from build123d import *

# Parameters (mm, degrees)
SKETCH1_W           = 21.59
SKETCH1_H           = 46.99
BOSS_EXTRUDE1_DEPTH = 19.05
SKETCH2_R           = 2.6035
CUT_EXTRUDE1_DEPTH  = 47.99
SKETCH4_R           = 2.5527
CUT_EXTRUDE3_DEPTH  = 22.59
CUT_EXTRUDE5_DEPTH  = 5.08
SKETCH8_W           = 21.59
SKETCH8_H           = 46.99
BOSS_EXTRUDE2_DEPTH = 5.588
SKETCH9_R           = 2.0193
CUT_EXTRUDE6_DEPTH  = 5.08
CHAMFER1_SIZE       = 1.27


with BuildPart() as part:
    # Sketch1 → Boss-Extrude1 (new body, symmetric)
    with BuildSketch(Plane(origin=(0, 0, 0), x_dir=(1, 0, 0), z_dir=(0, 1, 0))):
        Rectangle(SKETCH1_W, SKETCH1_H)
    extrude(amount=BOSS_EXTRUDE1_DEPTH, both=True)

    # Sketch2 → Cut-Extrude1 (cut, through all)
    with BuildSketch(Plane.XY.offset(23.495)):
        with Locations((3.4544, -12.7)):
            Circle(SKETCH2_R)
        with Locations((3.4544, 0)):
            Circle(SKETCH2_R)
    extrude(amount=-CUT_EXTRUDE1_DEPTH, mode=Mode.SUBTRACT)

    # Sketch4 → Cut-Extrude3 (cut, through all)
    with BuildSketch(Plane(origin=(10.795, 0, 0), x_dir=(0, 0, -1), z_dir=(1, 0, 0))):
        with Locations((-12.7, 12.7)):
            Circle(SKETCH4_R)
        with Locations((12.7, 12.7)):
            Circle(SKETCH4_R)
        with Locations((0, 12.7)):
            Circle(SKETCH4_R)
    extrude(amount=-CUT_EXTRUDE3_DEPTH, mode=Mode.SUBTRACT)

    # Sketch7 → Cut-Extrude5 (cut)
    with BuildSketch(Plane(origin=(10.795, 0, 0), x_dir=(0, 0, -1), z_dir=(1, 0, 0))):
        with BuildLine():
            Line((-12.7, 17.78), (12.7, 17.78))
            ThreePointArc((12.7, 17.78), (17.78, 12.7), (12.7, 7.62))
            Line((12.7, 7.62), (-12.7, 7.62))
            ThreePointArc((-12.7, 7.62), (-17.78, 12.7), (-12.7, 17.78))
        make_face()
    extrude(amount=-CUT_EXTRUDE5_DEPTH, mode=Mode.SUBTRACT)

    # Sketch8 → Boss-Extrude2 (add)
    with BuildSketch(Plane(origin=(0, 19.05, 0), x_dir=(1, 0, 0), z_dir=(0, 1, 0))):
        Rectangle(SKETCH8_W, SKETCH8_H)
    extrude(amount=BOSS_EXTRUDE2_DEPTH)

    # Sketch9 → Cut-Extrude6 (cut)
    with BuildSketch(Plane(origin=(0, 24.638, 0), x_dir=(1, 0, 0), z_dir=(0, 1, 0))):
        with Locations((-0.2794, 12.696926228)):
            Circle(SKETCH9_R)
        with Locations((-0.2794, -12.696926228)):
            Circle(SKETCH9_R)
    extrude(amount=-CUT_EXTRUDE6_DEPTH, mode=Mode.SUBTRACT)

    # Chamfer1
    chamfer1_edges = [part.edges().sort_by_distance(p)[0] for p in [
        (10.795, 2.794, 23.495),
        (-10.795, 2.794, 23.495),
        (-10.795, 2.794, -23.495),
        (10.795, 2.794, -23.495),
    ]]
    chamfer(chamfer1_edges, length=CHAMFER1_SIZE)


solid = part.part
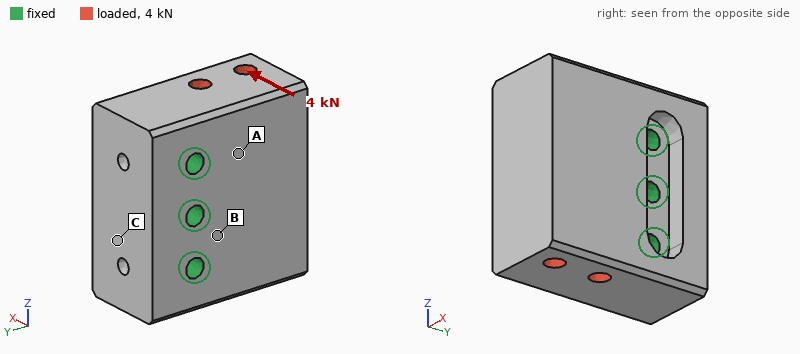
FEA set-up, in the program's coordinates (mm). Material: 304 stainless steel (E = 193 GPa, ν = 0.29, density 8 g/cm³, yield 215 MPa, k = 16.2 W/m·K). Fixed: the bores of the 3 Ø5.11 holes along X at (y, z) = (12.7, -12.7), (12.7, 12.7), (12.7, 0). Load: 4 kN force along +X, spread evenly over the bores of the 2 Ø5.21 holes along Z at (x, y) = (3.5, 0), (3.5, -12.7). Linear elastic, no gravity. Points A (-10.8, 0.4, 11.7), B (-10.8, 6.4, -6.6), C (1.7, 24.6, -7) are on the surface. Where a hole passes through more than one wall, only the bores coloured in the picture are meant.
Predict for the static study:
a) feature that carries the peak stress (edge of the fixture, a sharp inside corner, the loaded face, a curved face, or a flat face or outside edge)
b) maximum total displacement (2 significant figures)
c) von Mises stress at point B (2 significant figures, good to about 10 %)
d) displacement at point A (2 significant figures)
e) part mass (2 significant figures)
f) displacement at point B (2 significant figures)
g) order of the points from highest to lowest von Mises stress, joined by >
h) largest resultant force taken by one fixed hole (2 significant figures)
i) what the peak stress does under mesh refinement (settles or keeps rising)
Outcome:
edge of the fixture
7.1 µm
18 MPa
2.6 µm
310 g
1.3 µm
B > A > C
1.4 kN
keeps rising
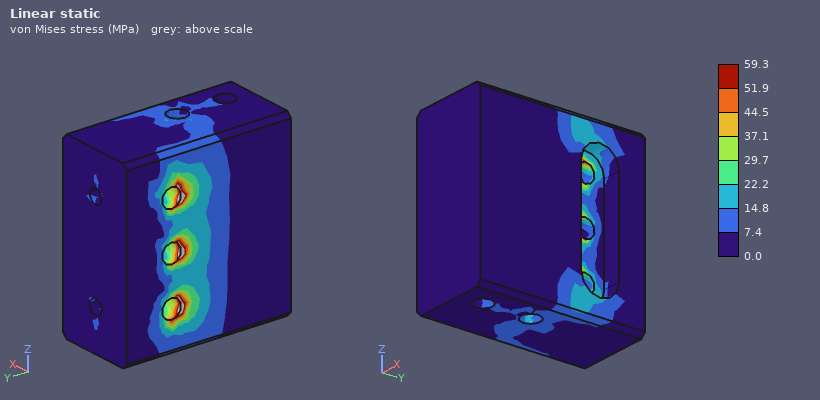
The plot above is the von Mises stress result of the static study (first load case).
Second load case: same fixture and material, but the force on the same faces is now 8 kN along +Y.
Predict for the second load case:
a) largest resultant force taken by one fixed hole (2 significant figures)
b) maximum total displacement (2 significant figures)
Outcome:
3.0 kN
5.1 µm
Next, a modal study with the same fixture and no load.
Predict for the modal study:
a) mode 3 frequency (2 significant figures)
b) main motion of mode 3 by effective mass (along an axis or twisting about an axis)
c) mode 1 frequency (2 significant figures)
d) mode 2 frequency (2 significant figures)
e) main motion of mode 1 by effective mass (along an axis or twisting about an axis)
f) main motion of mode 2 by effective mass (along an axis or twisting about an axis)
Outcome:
17 kHz
twisting about Y
10 kHz
15 kHz
along X
along Z
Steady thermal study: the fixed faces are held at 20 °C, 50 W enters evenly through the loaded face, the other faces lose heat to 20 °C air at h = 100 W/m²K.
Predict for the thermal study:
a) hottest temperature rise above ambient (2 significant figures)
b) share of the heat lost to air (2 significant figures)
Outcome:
51 K
35 %
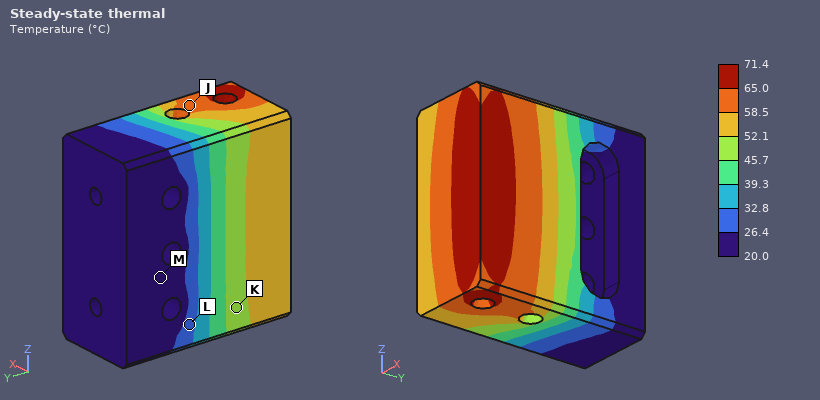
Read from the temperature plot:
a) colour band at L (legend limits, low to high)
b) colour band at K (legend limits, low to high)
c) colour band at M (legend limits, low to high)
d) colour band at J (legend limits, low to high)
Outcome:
26.4 to 32.8 °C
45.7 to 52.1 °C
20.0 to 26.4 °C
58.5 to 65.0 °C
